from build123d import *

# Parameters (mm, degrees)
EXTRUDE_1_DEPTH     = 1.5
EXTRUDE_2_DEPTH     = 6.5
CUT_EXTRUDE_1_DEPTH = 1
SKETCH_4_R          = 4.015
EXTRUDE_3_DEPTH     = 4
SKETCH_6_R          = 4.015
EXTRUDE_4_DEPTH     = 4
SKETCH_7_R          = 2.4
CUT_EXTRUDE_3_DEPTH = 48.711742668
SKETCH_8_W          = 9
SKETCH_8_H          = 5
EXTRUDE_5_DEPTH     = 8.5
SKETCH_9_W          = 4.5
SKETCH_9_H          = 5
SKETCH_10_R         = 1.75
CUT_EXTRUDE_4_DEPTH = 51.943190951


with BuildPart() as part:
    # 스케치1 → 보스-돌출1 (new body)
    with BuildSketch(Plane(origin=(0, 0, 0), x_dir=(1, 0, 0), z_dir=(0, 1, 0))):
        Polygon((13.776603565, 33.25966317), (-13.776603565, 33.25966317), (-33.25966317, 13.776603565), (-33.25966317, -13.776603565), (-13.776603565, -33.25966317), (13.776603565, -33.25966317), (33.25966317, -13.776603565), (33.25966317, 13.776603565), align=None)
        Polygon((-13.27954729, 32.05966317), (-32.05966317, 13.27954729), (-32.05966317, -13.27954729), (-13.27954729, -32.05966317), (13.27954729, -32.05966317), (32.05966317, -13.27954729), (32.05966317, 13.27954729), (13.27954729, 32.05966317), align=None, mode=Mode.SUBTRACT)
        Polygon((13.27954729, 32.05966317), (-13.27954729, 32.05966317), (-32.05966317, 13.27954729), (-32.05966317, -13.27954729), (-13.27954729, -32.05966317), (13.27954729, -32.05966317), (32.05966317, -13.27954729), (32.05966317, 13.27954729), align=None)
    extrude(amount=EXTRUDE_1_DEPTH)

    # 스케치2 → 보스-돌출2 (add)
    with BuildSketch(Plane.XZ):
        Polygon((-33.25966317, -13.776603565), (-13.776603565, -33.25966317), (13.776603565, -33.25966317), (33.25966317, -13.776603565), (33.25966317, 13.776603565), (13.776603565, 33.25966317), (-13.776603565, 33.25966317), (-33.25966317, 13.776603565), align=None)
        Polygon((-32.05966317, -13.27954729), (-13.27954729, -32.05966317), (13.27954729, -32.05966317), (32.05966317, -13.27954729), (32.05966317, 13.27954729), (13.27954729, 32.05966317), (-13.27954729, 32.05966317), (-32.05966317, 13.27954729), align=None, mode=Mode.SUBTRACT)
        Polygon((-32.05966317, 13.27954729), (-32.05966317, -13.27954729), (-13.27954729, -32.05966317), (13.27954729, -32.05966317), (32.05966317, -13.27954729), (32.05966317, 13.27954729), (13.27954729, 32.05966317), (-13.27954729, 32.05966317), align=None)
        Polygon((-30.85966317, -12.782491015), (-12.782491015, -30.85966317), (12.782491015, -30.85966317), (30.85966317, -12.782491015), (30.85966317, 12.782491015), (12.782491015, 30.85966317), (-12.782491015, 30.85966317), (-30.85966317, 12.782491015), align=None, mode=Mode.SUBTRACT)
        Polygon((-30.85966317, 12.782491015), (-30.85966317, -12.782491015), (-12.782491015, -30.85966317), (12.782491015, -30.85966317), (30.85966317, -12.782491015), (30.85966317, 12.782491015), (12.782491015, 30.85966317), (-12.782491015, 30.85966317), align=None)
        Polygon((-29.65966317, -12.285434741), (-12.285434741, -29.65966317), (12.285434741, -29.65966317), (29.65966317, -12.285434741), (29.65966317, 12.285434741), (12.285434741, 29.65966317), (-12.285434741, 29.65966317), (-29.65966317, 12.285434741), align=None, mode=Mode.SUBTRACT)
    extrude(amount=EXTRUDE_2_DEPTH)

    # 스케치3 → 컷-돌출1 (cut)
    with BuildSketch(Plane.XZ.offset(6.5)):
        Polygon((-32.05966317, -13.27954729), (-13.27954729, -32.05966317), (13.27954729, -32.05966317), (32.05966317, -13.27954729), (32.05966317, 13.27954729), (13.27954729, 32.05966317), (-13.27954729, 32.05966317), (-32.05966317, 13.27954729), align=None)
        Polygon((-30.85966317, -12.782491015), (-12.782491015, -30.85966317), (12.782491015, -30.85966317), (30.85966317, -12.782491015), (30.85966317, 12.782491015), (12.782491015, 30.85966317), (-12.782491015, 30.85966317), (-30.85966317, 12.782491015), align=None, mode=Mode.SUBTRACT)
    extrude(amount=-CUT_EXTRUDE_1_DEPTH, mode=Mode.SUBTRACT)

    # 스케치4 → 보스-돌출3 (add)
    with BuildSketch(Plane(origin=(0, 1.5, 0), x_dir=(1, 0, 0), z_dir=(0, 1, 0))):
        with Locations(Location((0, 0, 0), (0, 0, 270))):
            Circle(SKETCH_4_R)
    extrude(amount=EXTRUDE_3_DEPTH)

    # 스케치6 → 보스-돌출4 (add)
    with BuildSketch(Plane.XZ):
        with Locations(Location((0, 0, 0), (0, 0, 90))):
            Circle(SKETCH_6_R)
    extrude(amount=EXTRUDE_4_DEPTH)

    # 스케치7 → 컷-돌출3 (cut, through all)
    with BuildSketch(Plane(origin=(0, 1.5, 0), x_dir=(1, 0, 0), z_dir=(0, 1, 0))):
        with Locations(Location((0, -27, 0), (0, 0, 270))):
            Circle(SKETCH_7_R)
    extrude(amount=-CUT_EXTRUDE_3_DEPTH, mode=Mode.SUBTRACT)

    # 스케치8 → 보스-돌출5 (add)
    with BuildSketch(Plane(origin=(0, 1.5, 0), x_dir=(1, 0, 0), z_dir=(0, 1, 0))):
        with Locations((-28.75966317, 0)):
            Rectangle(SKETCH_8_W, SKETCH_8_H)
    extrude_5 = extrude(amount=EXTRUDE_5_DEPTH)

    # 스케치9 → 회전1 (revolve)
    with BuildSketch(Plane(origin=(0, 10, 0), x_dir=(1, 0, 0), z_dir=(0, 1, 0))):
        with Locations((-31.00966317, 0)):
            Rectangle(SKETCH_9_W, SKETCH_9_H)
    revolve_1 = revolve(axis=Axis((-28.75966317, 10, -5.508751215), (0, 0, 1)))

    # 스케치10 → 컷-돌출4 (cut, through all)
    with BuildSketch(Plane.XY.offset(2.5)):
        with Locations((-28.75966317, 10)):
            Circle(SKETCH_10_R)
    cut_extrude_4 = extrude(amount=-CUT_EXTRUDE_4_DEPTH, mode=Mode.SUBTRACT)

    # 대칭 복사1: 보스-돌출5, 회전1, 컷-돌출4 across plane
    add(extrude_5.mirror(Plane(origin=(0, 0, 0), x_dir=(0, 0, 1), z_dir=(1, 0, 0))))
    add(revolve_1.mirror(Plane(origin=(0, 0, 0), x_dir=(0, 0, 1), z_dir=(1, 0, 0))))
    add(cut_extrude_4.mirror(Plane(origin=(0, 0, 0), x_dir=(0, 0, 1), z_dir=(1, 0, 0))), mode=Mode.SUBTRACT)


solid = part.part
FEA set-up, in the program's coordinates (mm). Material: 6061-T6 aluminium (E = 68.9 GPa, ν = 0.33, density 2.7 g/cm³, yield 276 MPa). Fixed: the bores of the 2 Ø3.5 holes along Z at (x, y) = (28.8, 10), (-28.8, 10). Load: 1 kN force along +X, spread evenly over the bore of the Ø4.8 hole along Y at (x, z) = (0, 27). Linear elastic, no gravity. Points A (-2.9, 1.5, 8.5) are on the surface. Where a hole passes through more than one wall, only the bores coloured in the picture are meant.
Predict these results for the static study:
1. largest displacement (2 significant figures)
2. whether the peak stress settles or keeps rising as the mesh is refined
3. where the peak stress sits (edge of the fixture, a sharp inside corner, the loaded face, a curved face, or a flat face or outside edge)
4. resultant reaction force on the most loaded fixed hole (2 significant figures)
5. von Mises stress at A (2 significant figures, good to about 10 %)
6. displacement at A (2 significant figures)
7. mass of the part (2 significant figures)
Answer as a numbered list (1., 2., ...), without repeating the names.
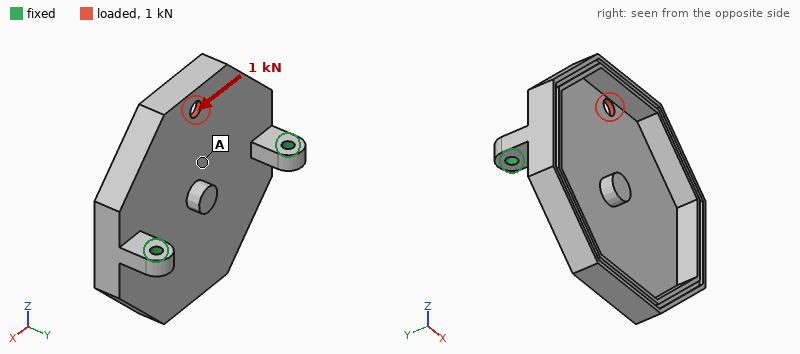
1. 53 µm
2. keeps rising
3. edge of the fixture
4. 680 N
5. 15 MPa
6. 25 µm
7. 31 g
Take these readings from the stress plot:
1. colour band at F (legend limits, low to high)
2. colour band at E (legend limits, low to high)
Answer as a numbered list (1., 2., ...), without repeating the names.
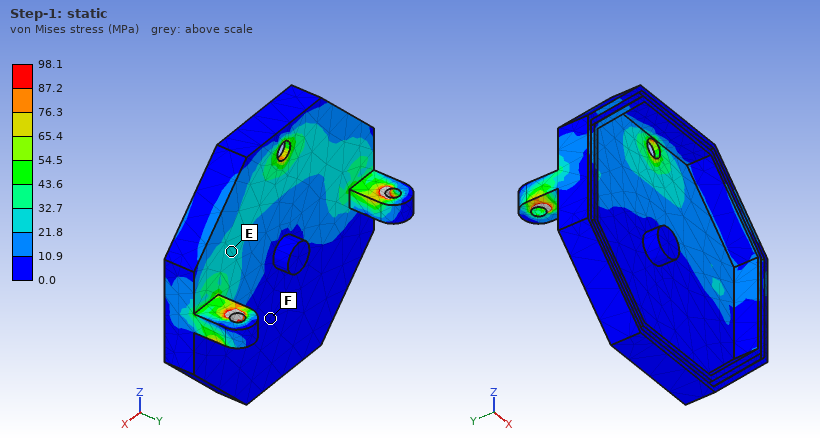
1. 0.0 to 10.9 MPa
2. 21.8 to 32.7 MPa
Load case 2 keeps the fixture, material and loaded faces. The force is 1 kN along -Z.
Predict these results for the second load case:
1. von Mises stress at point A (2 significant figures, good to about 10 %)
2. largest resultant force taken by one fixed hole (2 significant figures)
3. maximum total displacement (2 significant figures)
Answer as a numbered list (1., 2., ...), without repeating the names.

1. 16 MPa
2. 500 N
3. 0.10 mm
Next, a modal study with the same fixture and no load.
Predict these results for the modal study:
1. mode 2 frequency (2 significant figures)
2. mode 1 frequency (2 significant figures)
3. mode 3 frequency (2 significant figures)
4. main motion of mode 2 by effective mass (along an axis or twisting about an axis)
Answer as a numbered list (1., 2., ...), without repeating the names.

1. 2500 Hz
2. 1400 Hz
3. 3900 Hz
4. along Y
